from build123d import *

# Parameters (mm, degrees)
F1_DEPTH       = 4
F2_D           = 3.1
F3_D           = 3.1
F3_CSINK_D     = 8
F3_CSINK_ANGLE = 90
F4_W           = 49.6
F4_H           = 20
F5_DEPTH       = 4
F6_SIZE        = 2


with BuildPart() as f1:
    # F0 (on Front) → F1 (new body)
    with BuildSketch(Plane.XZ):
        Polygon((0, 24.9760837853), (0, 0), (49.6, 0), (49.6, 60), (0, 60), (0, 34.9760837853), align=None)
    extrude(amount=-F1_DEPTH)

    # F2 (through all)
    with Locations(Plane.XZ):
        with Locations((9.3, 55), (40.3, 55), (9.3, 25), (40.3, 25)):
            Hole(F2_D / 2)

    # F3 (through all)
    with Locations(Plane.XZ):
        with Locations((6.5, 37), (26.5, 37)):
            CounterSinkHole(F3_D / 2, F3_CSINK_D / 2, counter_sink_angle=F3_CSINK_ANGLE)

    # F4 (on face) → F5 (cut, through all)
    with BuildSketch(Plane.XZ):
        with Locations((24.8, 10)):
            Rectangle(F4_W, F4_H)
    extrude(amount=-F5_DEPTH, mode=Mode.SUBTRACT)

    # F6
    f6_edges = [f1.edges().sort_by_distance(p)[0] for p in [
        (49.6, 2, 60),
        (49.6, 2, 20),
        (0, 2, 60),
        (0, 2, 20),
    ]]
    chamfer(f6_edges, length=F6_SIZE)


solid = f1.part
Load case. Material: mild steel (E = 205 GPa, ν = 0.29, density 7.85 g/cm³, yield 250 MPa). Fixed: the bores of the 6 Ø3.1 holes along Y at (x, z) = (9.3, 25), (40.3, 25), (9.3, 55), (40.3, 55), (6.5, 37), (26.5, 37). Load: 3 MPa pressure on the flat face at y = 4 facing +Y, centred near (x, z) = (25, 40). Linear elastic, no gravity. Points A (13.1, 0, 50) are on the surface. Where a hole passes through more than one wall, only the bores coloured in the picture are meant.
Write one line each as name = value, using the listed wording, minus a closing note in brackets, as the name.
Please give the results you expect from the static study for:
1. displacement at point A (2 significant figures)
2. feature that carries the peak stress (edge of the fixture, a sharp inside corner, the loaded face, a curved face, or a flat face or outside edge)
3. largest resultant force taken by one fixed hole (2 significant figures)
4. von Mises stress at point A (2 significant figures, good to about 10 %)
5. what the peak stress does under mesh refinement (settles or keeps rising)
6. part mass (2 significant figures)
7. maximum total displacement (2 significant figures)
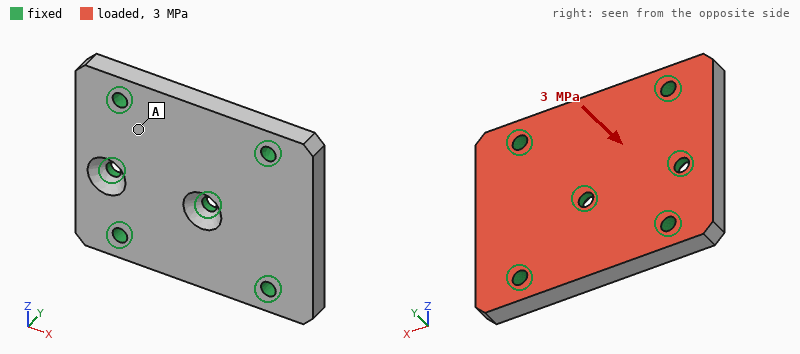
displacement at point A = 2.4 µm
feature that carries the peak stress = edge of the fixture
largest resultant force taken by one fixed hole = 1.2 kN
von Mises stress at point A = 23 MPa
what the peak stress does under mesh refinement = keeps rising
part mass = 60 g
maximum total displacement = 10 µm
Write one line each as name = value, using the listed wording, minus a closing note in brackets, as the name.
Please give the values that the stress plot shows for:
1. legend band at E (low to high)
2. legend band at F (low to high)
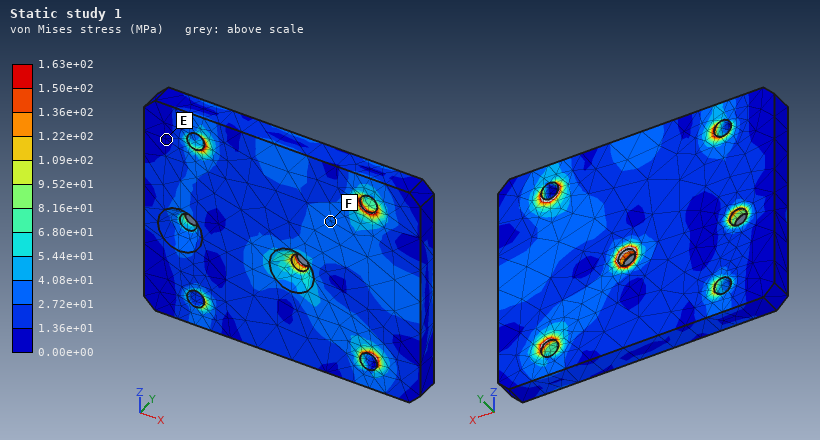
legend band at E = 0.00e+00 to 1.36e+01 MPa
legend band at F = 2.72e+01 to 4.08e+01 MPa
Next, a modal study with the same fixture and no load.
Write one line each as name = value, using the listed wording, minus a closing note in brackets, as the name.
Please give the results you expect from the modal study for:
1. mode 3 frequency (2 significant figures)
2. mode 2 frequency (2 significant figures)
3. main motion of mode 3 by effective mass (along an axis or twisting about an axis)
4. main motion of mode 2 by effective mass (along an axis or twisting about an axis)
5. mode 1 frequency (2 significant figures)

mode 3 frequency = 25 kHz
mode 2 frequency = 22 kHz
main motion of mode 3 by effective mass = along Y
main motion of mode 2 by effective mass = along Y
mode 1 frequency = 19 kHz
